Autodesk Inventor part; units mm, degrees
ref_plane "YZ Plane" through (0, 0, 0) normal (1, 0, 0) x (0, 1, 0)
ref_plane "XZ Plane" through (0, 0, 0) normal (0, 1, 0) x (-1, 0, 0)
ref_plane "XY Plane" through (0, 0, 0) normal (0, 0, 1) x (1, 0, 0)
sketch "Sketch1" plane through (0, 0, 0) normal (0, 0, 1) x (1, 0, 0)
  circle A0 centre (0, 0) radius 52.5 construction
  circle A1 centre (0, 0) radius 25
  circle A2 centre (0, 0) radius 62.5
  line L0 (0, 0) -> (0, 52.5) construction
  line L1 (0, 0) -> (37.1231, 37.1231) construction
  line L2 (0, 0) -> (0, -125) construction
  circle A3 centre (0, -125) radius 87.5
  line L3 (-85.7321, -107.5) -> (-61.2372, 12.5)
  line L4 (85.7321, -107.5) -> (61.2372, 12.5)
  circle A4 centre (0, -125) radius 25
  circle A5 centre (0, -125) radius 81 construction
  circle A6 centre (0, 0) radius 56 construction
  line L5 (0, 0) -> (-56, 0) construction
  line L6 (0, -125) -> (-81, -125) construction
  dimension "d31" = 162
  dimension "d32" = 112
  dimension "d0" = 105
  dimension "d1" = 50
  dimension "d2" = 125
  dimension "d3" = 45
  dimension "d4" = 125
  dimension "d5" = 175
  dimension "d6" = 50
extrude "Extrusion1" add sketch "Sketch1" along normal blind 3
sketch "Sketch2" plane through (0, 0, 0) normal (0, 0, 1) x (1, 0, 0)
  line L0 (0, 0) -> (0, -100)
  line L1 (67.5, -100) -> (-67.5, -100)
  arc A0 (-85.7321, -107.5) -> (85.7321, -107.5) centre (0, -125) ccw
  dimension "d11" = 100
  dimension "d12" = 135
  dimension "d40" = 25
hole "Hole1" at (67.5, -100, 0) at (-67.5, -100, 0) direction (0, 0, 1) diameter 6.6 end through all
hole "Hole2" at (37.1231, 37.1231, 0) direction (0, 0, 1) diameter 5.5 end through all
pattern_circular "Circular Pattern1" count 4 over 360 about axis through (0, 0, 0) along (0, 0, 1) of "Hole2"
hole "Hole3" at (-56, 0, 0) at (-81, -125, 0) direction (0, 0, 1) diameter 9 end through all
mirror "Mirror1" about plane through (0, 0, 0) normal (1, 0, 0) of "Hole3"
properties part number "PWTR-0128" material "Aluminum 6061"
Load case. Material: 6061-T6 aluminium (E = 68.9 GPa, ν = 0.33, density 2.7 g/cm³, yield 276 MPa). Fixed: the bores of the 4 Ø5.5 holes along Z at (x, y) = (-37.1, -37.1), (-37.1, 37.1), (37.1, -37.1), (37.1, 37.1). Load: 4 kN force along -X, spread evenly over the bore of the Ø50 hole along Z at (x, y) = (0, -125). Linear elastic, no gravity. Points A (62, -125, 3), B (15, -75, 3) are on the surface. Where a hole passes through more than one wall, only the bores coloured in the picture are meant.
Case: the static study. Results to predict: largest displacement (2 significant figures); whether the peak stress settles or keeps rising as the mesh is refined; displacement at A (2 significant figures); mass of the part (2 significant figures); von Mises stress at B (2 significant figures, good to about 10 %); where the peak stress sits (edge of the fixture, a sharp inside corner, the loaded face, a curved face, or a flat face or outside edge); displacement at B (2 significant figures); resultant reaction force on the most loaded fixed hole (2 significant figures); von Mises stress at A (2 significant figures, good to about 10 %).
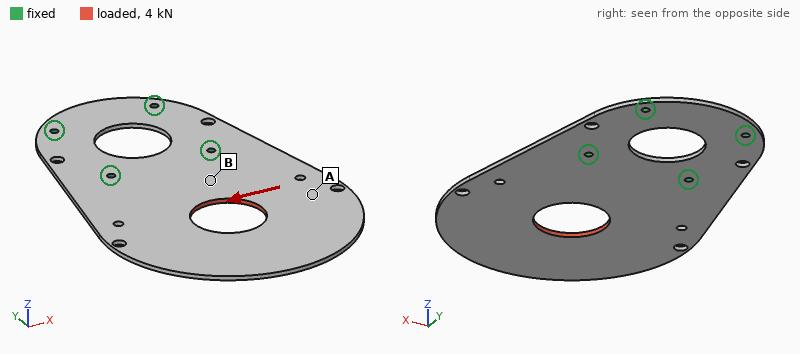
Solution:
0.15 mm
keeps rising
0.096 mm
270 g
29 MPa
edge of the fixture
0.035 mm
3.9 kN
9.2 MPa
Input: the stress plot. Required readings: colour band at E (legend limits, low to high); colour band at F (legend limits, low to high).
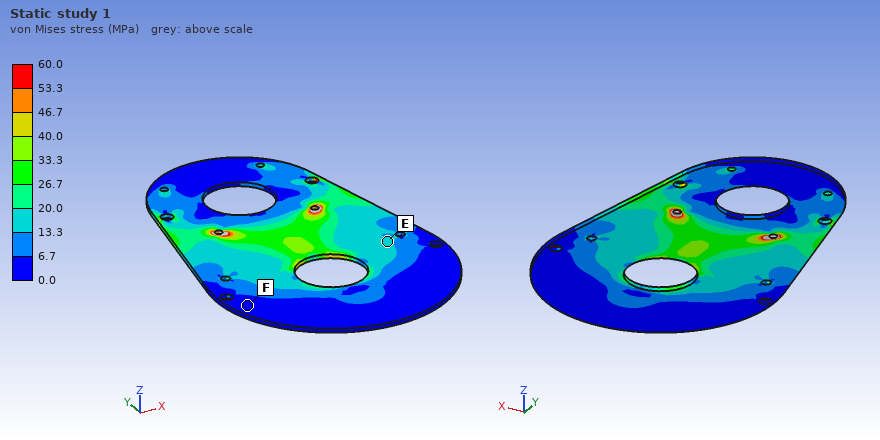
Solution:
13.3 to 20.0 MPa
0.0 to 6.7 MPa
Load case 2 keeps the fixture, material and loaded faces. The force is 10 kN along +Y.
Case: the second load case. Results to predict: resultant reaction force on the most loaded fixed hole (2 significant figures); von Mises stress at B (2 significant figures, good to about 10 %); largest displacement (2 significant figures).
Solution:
4.2 kN
25 MPa
65 µm
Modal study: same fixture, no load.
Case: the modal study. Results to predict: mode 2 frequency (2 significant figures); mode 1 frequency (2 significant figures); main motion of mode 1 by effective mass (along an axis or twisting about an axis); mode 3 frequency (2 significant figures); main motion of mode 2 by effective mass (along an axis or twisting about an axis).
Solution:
220 Hz
87 Hz
along Z
460 Hz
twisting about Y
